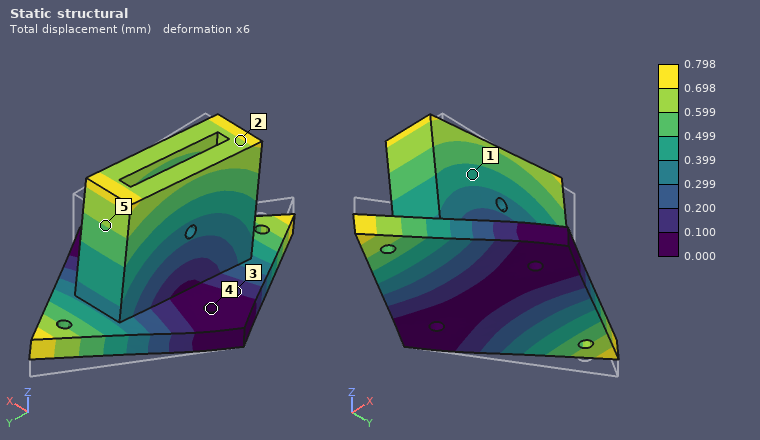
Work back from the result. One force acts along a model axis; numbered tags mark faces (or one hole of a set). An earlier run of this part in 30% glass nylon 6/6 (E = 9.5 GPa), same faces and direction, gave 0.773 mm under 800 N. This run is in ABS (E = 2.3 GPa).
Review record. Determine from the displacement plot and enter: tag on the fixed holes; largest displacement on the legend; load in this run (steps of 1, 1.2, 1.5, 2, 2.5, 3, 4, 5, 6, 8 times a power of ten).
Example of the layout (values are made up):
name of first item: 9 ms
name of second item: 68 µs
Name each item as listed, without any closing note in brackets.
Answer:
tag on the fixed holes: 4
largest displacement on the legend: 0.798 mm
load in this run: 200 N
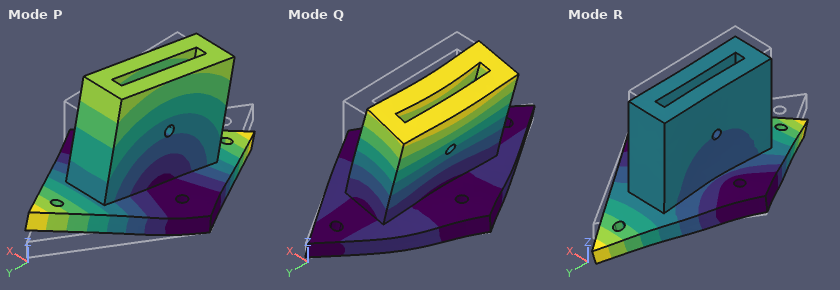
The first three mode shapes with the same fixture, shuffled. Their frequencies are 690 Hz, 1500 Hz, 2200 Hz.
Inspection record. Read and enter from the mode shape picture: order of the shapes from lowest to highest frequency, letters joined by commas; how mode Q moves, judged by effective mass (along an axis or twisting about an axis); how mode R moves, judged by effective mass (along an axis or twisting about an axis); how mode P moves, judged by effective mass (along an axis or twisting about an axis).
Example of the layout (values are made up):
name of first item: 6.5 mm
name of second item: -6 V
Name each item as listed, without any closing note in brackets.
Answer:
order of the shapes from lowest to highest frequency, letters joined by commas: P, Q, R
how mode Q moves, judged by effective mass: along X
how mode R moves, judged by effective mass: along Z
how mode P moves, judged by effective mass: along Y
